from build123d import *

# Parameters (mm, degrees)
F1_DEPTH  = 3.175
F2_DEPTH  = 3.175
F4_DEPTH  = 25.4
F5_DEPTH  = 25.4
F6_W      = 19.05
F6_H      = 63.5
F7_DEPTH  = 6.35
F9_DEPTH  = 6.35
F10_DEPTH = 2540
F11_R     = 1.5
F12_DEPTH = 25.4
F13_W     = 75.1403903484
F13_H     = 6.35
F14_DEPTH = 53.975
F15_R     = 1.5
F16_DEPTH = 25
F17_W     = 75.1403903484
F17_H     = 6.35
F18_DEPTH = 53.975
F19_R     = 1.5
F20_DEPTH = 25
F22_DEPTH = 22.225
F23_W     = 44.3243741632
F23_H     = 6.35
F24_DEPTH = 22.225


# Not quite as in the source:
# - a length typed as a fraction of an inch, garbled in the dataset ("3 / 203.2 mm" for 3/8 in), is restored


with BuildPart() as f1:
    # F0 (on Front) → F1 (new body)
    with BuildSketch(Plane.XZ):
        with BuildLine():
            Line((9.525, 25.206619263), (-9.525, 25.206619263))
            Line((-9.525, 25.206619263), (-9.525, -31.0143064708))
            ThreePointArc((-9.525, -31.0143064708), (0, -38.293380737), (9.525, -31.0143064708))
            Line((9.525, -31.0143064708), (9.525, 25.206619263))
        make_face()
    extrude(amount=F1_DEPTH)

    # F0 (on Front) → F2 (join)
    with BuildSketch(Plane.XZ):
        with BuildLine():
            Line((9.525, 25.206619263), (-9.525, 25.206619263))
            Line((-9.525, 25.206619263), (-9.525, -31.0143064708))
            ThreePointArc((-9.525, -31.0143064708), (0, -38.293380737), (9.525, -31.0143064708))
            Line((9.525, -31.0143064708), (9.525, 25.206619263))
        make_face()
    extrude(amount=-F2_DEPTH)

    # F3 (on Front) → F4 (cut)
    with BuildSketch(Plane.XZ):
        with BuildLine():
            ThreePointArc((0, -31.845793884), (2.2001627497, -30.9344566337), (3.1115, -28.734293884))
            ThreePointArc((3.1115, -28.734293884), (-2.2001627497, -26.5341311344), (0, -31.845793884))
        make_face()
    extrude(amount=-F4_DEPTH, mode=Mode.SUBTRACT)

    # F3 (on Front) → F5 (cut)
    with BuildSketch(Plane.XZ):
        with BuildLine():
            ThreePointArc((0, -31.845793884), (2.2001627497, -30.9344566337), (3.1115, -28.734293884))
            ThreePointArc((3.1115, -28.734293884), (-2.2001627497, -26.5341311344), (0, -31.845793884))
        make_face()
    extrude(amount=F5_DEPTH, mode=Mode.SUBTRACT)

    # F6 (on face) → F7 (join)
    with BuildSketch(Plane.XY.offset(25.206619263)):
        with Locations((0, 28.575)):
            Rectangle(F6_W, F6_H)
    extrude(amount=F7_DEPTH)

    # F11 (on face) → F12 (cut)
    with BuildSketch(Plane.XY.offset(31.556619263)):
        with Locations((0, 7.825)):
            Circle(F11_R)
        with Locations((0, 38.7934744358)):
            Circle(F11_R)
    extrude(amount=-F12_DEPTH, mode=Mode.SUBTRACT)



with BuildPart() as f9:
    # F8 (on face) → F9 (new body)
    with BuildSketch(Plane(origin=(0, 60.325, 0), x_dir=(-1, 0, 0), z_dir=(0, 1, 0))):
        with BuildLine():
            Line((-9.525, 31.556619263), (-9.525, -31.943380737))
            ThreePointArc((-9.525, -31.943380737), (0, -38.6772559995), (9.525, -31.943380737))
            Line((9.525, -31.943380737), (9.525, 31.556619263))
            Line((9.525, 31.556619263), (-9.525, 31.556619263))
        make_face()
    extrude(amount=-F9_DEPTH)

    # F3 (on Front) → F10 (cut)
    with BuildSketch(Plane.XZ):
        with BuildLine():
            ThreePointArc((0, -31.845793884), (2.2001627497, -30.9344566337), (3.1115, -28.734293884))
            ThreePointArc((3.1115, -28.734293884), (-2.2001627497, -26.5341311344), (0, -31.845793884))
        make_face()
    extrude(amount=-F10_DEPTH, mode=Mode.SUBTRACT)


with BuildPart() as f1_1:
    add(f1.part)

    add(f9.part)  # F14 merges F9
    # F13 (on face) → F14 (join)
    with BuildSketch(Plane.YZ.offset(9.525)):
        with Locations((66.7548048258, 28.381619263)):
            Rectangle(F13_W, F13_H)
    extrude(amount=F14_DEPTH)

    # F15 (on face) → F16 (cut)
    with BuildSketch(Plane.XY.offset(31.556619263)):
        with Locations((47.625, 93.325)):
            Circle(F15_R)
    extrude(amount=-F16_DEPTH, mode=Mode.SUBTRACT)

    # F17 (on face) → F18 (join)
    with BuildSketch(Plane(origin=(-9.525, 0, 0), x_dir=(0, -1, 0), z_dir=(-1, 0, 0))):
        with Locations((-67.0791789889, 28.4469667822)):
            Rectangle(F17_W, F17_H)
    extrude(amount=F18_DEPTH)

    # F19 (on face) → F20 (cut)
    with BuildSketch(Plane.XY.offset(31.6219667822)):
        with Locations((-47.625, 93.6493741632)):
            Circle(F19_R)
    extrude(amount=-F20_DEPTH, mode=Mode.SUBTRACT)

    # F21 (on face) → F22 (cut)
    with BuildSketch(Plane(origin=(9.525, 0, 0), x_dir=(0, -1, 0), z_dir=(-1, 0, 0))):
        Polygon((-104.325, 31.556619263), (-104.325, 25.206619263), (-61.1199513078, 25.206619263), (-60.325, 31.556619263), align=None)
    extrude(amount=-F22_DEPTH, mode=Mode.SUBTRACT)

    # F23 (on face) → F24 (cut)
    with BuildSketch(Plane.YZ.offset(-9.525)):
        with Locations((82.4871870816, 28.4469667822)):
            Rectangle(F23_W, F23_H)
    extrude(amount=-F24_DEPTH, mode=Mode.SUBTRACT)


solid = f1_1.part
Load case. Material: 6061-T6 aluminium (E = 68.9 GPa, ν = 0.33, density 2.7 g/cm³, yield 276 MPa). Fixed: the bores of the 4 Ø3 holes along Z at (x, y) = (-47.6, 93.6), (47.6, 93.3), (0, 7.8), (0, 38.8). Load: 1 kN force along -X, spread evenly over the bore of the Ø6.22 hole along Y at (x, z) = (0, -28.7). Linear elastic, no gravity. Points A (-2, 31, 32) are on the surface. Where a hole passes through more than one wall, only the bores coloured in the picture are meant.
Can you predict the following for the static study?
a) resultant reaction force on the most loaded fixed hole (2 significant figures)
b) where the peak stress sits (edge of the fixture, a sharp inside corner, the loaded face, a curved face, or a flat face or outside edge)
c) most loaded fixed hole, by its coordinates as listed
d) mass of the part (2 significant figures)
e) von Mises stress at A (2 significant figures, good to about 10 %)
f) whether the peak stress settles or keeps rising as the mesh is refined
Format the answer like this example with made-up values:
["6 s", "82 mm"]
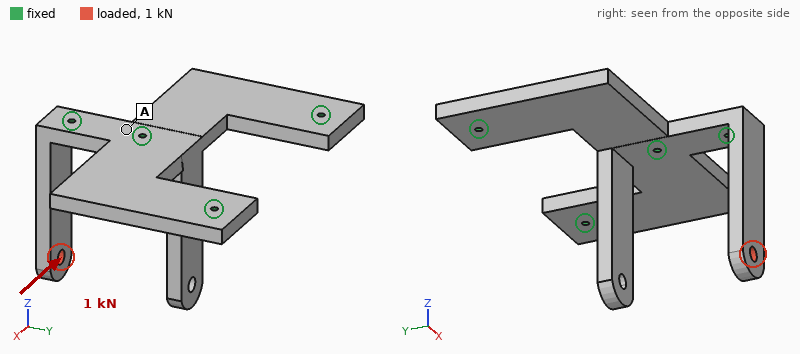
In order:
["1.2 kN", "edge of the fixture", "(0, 7.8)", "170 g", "31 MPa", "keeps rising"]
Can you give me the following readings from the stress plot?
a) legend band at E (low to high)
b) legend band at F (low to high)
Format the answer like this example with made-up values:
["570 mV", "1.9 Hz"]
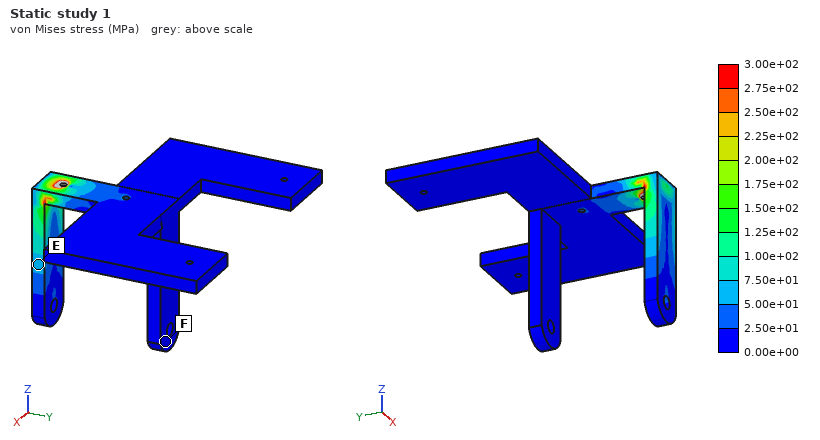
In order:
["5.00e+01 to 7.50e+01 MPa", "0.00e+00 to 2.50e+01 MPa"]
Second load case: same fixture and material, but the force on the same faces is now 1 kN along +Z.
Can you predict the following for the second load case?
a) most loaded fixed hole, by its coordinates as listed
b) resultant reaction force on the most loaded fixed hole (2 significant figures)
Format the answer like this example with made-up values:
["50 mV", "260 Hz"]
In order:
["(0, 7.8)", "1.1 kN"]
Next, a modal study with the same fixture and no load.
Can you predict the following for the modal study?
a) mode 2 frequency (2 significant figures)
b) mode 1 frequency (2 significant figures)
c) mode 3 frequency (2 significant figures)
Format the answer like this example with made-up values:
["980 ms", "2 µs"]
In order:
["1100 Hz", "1000 Hz", "1800 Hz"]
